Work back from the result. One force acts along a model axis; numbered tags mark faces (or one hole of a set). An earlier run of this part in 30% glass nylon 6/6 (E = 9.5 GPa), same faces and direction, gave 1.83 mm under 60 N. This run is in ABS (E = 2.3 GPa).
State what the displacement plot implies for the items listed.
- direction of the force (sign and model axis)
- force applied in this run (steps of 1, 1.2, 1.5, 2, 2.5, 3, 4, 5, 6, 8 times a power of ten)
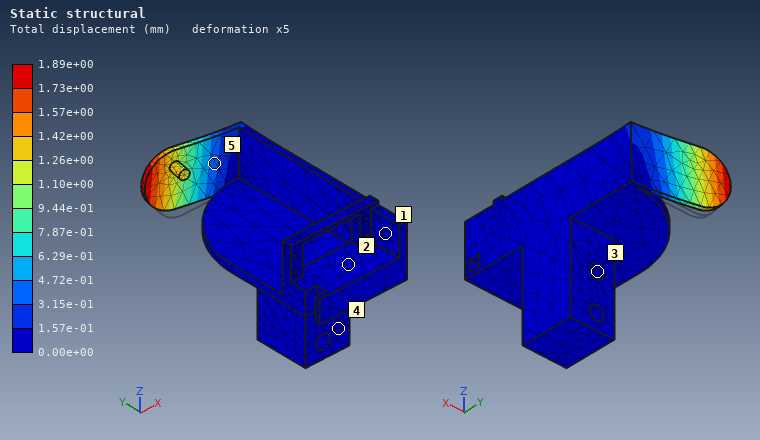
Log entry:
+Y
15 N
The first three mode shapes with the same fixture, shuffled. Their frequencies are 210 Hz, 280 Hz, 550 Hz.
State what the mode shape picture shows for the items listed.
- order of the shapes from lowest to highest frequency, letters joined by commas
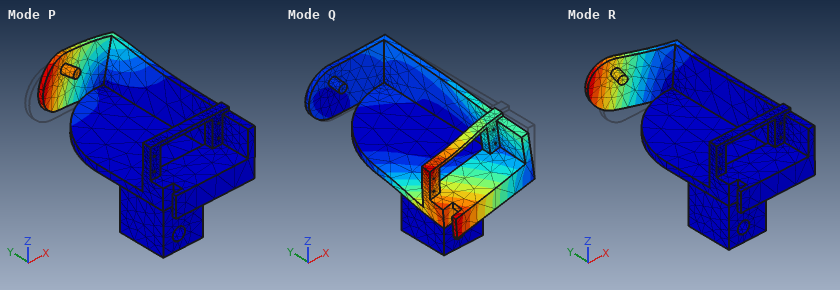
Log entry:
R, P, Q
